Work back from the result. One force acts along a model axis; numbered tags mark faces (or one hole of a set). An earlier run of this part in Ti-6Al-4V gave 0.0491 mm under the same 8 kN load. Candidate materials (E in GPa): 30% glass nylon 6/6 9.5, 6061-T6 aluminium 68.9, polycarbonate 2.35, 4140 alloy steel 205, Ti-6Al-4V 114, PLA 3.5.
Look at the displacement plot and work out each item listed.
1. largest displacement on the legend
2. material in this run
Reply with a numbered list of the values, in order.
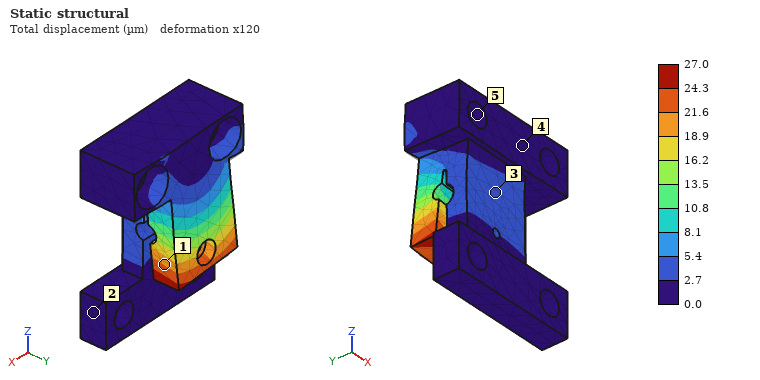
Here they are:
1. 27.0 µm
2. 4140 alloy steel
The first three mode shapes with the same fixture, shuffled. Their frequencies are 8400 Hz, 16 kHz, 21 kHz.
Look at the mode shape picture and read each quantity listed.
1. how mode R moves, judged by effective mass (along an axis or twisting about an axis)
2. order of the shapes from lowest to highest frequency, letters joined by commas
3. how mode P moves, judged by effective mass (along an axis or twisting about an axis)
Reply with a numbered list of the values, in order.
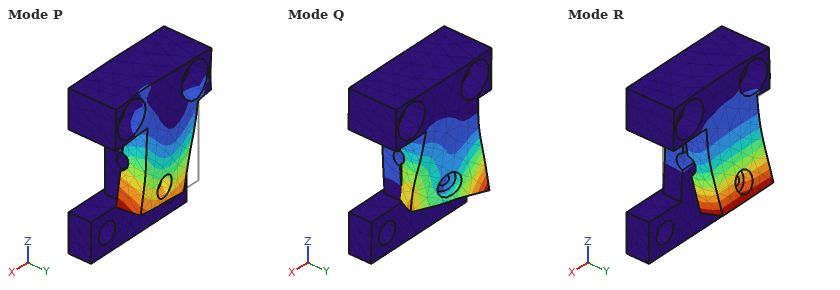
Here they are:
1. along Y
2. R, P, Q
3. along X
